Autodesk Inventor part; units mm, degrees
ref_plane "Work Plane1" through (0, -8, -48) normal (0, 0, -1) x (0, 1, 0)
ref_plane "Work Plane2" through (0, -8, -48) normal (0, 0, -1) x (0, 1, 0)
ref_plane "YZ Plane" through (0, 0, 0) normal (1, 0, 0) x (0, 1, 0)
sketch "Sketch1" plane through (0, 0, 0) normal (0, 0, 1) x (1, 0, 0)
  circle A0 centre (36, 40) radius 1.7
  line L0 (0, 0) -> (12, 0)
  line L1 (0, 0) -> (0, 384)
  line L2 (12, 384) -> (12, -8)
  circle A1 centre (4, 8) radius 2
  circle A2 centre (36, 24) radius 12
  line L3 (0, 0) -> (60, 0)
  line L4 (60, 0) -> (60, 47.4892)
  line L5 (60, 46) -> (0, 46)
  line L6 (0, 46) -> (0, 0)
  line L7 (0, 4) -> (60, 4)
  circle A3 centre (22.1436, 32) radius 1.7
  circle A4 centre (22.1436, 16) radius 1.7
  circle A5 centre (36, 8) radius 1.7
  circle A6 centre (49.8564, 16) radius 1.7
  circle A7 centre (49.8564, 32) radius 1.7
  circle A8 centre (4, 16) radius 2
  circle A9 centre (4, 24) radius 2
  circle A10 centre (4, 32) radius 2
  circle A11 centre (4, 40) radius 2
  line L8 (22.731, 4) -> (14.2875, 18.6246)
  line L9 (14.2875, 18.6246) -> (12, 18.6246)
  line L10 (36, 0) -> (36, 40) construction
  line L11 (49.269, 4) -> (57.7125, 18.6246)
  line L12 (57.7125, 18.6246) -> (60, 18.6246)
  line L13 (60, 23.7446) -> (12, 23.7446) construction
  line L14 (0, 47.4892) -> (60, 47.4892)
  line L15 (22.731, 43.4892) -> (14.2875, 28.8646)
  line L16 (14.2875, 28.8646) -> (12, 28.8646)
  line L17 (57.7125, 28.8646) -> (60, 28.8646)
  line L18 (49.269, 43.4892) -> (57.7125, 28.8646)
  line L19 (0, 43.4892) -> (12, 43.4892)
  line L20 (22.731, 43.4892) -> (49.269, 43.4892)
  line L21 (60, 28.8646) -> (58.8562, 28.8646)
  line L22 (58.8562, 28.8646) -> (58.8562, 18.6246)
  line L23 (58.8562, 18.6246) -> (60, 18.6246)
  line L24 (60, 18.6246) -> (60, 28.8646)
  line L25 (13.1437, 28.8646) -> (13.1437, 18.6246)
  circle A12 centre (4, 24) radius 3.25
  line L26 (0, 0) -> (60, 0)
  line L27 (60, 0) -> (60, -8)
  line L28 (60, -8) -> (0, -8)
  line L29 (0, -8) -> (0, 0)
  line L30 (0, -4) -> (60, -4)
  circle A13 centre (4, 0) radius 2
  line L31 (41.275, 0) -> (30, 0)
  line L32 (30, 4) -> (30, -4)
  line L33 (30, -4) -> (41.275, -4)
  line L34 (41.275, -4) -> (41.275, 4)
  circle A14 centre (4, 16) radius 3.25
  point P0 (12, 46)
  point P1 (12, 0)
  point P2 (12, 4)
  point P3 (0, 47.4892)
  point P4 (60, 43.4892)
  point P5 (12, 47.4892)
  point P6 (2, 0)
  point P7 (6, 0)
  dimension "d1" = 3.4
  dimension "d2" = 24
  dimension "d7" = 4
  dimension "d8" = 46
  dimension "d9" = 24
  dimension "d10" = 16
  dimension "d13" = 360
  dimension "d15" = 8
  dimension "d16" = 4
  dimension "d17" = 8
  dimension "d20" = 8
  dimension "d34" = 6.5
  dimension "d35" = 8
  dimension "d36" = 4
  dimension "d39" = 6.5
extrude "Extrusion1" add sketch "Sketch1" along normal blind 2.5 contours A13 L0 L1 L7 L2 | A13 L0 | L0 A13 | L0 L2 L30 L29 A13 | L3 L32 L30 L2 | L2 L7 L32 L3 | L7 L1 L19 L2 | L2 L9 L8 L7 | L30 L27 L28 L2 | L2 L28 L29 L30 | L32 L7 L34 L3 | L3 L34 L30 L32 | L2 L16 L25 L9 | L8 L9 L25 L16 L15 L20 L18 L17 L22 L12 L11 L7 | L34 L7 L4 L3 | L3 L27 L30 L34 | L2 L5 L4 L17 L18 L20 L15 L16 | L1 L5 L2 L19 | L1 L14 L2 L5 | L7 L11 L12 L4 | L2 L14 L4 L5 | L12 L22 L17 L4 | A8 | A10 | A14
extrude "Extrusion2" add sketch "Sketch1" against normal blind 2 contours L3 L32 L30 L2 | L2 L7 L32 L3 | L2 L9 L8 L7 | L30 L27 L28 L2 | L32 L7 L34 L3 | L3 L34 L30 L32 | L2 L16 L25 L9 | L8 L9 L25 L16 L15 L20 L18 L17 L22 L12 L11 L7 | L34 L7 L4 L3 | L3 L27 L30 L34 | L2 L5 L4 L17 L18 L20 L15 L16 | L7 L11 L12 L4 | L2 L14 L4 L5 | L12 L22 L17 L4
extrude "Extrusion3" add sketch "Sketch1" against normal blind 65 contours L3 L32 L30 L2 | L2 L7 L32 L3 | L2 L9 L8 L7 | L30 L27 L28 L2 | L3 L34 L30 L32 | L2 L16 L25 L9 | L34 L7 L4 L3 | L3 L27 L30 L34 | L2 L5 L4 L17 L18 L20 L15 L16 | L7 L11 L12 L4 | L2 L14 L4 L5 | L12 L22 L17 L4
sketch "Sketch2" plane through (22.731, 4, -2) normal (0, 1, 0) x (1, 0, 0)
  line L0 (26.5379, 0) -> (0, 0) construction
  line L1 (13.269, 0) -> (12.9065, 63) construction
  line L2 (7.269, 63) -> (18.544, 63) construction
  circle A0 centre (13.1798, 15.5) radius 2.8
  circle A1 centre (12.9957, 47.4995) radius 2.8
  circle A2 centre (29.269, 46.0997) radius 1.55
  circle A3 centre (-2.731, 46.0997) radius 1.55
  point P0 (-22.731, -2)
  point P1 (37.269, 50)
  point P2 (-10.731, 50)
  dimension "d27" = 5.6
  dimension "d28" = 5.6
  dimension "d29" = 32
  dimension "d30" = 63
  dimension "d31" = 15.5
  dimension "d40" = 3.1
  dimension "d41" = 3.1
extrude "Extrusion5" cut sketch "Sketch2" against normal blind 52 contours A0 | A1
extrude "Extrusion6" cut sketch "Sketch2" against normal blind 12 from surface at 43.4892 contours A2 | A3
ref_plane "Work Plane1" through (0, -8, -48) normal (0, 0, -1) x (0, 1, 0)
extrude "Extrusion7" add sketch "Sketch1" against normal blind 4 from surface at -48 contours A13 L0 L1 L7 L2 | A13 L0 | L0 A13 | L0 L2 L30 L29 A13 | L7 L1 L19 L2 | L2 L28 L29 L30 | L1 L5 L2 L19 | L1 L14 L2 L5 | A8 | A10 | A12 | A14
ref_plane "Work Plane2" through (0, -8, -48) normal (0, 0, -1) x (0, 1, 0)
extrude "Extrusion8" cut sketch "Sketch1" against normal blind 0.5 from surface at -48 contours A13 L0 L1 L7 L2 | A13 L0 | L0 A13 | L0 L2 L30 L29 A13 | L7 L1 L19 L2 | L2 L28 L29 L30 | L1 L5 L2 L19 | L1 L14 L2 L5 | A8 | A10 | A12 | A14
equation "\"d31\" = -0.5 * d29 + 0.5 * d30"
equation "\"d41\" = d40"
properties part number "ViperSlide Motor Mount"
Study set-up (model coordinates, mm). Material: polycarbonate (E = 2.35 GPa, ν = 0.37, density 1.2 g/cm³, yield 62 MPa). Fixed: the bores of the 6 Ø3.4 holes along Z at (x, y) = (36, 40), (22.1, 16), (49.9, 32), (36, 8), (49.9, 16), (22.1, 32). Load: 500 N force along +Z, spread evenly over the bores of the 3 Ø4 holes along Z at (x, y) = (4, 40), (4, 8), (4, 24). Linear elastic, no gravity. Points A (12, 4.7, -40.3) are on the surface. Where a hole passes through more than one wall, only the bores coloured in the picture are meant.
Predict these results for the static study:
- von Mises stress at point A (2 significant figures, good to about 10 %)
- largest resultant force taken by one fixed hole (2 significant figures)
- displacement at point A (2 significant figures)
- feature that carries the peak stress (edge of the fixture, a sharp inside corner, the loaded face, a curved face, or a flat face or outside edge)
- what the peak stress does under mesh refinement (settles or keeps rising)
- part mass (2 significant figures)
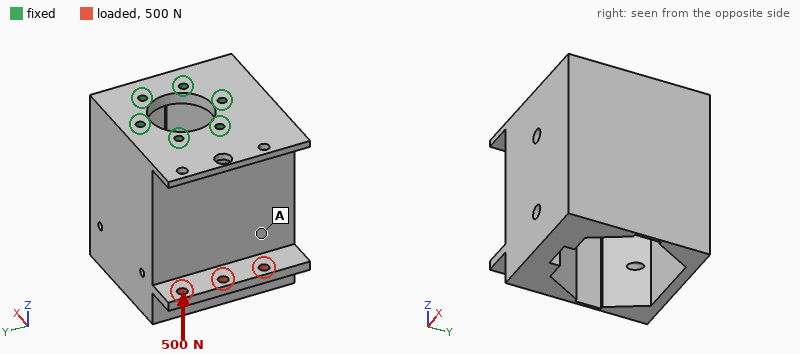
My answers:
3.3 MPa
300 N
0.27 mm
edge of the fixture
keeps rising
100 g
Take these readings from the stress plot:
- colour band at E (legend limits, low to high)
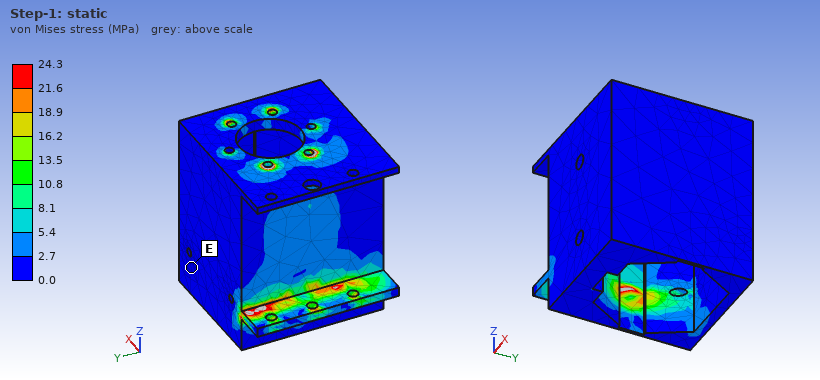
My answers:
0.0 to 2.7 MPa
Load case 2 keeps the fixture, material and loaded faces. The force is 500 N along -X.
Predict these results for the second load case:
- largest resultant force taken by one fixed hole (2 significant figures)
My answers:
370 N
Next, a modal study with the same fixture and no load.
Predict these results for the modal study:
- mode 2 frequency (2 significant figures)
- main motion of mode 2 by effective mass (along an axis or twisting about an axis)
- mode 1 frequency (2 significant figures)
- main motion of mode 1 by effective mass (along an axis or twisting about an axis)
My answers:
650 Hz
along X
610 Hz
along Y
